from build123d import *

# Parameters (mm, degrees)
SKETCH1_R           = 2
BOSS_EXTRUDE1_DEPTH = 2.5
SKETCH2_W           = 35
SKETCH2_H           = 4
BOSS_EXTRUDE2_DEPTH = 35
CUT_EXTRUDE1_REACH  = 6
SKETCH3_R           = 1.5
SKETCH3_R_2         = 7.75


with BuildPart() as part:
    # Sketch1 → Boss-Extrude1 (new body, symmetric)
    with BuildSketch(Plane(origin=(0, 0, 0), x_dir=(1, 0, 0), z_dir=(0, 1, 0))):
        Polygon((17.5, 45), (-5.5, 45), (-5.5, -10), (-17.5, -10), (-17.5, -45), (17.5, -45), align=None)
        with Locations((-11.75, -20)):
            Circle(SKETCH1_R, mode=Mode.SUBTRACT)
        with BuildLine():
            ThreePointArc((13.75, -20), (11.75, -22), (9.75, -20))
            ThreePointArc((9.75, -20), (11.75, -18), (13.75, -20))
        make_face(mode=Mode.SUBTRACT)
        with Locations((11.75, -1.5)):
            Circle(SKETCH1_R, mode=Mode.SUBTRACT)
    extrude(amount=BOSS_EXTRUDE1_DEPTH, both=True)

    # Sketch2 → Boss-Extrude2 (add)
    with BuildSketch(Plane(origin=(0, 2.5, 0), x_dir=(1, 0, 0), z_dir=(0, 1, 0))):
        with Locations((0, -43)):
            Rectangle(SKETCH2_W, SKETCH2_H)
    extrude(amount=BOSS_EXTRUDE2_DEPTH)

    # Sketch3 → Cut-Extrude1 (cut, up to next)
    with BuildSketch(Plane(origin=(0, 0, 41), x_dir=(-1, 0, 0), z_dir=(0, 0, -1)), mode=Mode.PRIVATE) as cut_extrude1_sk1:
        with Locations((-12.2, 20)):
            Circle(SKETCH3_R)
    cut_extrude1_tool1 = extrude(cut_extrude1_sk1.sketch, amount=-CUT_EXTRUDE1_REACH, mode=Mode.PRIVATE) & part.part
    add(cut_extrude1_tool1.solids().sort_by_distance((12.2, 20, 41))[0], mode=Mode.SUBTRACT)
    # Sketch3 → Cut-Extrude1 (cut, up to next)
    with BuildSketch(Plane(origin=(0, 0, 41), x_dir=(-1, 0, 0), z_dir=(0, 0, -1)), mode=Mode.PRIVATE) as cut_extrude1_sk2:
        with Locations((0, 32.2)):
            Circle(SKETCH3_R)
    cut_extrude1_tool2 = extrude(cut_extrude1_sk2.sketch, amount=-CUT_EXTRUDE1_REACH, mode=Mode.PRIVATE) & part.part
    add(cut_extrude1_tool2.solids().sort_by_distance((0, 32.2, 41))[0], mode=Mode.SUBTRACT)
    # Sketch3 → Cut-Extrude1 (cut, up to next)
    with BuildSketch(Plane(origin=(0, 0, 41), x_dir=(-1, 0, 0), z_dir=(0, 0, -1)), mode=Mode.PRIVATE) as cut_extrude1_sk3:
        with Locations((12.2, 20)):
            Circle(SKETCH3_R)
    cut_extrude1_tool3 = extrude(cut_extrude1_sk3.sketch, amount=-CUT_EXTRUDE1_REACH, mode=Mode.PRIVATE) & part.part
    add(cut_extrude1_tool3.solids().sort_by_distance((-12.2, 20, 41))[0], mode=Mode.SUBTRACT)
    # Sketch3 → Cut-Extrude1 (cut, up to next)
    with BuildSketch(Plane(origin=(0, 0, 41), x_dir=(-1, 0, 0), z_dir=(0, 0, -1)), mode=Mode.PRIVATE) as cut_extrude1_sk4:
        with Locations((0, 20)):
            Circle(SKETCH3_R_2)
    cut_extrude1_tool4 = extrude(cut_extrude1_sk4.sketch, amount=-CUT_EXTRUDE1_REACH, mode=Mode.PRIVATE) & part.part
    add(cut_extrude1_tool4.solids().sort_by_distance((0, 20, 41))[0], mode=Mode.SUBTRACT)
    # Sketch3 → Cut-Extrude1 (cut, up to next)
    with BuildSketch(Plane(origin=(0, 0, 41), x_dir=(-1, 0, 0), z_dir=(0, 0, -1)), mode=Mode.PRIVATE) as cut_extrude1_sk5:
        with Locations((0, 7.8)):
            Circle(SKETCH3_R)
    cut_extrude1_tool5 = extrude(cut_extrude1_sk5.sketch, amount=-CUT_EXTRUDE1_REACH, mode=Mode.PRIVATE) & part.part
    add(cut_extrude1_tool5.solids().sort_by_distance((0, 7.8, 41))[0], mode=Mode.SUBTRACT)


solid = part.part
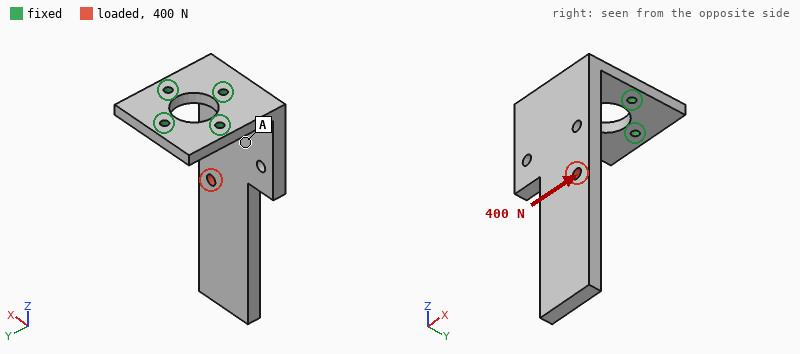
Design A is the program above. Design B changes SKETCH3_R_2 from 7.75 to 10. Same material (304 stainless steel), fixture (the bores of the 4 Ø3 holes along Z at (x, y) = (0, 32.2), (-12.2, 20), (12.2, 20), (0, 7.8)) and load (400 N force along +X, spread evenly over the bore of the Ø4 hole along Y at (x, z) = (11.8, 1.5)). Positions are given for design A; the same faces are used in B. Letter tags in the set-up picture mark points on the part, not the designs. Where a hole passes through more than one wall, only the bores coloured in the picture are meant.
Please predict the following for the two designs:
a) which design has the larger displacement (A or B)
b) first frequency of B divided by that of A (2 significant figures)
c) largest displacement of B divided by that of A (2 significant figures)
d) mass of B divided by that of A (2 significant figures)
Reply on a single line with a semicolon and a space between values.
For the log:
B; 0.99; 1.1; 0.97
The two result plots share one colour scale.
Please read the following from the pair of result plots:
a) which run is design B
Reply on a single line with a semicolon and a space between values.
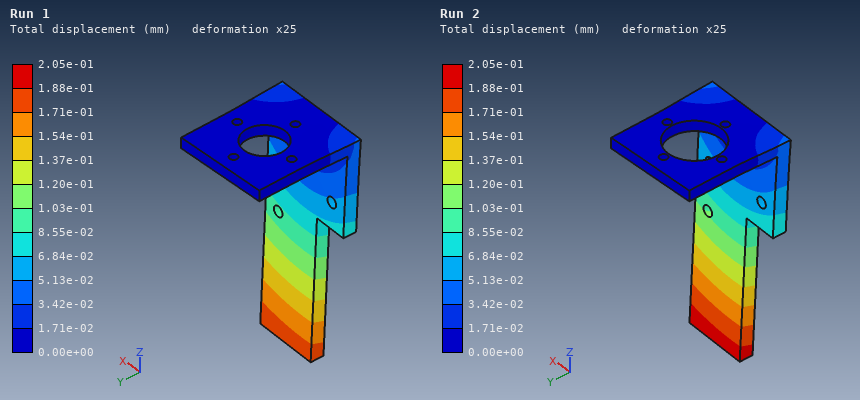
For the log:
Run 2
